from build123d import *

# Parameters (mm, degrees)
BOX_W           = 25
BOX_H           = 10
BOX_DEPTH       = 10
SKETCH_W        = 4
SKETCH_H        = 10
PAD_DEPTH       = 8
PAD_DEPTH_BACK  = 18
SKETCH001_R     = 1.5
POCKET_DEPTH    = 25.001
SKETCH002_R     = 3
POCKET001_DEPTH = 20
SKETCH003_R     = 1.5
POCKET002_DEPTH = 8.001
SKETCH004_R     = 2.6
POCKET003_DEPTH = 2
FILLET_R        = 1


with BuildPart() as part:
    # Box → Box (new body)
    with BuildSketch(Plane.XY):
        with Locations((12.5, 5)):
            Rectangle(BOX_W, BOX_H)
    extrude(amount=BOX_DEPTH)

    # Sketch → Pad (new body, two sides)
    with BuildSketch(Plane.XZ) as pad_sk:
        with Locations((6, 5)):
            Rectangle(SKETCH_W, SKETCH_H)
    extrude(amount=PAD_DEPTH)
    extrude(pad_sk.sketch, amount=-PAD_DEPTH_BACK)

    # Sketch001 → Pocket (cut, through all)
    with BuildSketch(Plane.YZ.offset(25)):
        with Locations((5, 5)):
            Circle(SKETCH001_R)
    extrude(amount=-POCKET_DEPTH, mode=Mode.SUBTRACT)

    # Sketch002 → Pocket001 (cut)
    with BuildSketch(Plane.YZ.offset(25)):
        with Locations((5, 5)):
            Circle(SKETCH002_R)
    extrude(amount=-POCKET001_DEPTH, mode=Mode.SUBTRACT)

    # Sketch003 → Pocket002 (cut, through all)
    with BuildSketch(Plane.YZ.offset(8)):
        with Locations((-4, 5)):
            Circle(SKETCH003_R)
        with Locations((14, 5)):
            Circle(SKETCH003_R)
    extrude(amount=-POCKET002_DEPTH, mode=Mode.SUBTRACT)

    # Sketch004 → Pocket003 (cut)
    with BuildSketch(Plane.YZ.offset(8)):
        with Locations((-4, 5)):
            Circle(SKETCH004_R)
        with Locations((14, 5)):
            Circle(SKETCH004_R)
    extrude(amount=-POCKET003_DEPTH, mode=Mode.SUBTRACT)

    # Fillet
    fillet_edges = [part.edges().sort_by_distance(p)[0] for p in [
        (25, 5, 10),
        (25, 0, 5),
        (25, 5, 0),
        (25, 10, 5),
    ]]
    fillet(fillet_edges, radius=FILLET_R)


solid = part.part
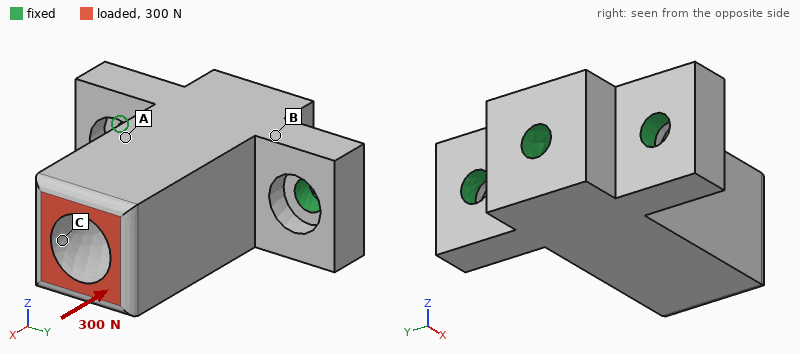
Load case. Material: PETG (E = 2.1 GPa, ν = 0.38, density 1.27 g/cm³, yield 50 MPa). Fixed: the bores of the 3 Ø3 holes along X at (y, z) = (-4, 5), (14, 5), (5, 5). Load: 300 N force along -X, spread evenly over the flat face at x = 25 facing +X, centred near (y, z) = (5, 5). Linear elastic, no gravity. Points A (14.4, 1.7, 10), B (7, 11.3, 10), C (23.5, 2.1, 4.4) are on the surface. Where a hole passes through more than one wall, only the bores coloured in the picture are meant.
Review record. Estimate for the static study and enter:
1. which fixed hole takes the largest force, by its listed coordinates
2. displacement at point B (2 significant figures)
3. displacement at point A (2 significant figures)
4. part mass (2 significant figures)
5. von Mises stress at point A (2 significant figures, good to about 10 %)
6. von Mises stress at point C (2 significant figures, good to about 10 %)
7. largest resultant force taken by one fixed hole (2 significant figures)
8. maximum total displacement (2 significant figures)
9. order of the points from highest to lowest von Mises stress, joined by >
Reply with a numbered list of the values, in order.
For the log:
1. (5, 5)
2. 13 µm
3. 31 µm
4. 3.1 g
5. 4.3 MPa
6. 8.2 MPa
7. 220 N
8. 59 µm
9. C > A > B
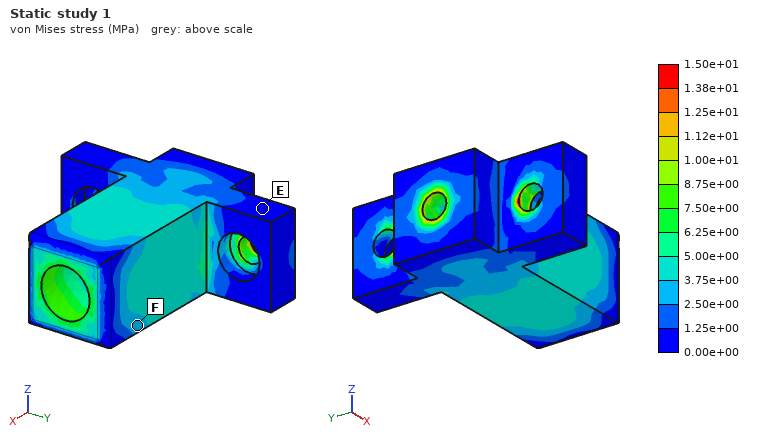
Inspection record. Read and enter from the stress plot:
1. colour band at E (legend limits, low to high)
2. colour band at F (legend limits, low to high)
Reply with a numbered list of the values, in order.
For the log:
1. 0.00e+00 to 1.25e+00 MPa
2. 2.50e+00 to 3.75e+00 MPa
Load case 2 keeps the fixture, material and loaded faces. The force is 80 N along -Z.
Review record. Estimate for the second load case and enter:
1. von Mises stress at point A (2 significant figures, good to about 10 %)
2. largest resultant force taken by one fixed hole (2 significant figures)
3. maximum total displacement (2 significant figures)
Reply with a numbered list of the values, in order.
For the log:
1. 5.6 MPa
2. 42 N
3. 0.39 mm
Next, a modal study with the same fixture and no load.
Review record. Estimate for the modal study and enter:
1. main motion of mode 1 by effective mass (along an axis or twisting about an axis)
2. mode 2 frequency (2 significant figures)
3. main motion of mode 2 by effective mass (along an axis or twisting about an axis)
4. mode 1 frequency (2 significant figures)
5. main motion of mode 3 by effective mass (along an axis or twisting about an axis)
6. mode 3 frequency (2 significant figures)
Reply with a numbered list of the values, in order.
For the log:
1. along Z
2. 4300 Hz
3. along Y
4. 3000 Hz
5. twisting about X
6. 9000 Hz
